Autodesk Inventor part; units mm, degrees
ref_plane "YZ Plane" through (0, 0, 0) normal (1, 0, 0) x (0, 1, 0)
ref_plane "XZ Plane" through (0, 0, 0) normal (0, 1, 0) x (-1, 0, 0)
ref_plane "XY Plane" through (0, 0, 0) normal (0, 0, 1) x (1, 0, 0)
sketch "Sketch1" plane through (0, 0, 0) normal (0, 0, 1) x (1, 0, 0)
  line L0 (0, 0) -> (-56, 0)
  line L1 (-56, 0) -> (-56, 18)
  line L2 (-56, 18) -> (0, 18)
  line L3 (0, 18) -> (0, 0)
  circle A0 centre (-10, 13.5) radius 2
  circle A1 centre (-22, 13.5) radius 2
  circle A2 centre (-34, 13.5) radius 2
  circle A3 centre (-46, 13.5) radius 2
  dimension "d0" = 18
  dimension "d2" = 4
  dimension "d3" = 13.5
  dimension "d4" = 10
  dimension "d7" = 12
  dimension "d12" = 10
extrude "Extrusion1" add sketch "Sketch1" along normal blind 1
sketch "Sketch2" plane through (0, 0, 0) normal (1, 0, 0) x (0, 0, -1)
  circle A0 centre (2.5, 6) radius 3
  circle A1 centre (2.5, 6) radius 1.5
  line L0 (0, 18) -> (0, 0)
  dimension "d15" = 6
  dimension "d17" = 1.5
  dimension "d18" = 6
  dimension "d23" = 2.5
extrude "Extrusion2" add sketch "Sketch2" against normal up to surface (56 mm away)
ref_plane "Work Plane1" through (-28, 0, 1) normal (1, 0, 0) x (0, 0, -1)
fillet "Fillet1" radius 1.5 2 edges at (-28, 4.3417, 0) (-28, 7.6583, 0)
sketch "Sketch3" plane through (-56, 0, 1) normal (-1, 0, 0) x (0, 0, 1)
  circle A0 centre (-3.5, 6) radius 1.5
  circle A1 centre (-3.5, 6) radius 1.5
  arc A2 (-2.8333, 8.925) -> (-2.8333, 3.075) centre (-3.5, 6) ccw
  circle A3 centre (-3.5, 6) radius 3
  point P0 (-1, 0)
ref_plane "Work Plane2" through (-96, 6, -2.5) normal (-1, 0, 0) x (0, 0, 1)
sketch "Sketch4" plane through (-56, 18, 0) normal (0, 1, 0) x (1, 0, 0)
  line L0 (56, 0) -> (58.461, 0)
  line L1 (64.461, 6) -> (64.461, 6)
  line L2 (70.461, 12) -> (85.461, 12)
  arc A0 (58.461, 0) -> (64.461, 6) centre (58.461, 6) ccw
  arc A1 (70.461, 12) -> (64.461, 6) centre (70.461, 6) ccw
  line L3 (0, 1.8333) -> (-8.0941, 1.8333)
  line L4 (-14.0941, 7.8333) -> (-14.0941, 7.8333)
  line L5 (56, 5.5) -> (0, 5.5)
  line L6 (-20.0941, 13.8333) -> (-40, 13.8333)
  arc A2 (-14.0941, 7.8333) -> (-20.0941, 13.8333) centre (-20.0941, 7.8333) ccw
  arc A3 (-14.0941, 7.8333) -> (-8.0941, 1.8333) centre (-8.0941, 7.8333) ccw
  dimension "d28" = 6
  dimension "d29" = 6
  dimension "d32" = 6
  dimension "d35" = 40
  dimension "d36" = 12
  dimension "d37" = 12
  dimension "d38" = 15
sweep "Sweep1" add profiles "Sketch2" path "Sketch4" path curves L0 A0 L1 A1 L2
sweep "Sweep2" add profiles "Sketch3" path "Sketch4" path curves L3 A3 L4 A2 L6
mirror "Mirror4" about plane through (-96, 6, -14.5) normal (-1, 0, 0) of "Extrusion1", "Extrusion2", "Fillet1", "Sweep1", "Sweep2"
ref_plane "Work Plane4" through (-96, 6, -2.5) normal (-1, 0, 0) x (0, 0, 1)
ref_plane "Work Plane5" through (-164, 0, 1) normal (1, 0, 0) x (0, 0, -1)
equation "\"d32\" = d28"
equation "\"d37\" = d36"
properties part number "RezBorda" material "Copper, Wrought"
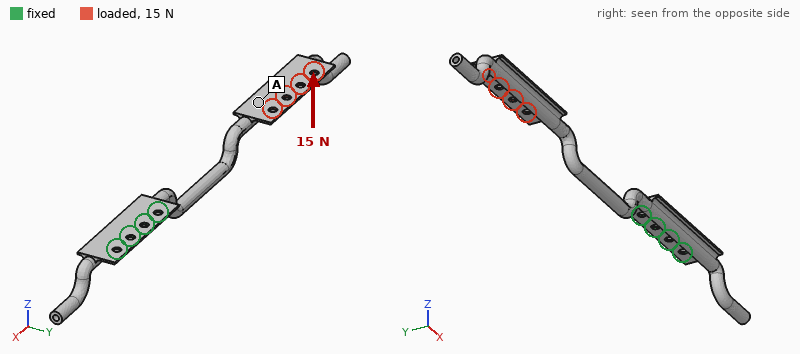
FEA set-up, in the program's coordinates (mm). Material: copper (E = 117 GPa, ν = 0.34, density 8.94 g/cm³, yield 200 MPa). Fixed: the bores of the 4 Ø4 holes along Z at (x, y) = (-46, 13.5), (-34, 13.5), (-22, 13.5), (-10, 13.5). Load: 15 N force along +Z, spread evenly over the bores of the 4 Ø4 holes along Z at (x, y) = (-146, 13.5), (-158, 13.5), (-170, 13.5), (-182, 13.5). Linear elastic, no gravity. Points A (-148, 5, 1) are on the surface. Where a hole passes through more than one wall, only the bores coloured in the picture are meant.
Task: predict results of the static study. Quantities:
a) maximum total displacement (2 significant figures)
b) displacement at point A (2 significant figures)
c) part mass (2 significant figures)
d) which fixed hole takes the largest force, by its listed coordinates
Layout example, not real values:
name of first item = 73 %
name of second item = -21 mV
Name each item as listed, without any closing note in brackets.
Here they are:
maximum total displacement = 2.4 mm
displacement at point A = 1.1 mm
part mass = 71 g
which fixed hole takes the largest force, by its listed coordinates = (-46, 13.5)
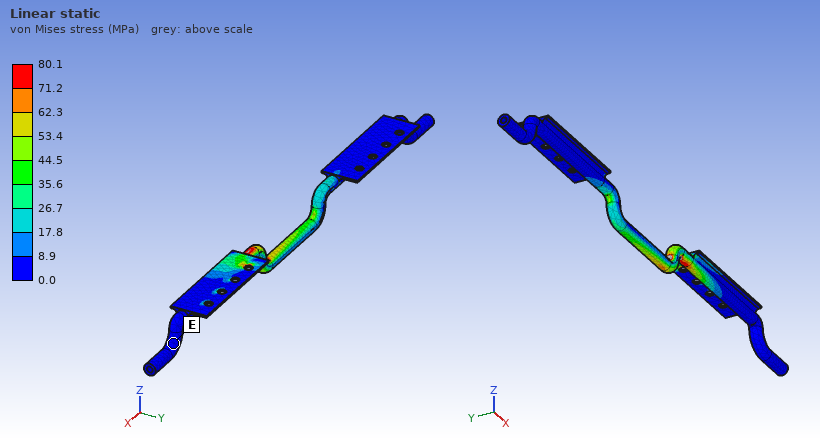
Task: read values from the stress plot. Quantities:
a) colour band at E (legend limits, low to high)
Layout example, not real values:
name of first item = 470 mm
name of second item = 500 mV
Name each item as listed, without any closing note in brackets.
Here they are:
colour band at E = 0.0 to 8.9 MPa
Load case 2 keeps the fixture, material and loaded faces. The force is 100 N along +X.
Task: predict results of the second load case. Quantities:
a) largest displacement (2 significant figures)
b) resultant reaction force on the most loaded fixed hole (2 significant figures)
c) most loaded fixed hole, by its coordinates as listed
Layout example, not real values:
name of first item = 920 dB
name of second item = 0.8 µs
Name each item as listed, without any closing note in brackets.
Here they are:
largest displacement = 2.4 mm
resultant reaction force on the most loaded fixed hole = 85 N
most loaded fixed hole, by its coordinates as listed = (-46, 13.5)
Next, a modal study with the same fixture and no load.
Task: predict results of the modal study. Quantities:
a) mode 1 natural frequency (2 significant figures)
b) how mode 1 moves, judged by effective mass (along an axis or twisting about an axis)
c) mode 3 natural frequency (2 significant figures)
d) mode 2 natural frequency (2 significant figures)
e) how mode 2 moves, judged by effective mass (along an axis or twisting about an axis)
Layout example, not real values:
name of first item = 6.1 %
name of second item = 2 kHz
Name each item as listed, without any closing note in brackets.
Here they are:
mode 1 natural frequency = 83 Hz
how mode 1 moves, judged by effective mass = along Z
mode 3 natural frequency = 570 Hz
mode 2 natural frequency = 87 Hz
how mode 2 moves, judged by effective mass = along Y
